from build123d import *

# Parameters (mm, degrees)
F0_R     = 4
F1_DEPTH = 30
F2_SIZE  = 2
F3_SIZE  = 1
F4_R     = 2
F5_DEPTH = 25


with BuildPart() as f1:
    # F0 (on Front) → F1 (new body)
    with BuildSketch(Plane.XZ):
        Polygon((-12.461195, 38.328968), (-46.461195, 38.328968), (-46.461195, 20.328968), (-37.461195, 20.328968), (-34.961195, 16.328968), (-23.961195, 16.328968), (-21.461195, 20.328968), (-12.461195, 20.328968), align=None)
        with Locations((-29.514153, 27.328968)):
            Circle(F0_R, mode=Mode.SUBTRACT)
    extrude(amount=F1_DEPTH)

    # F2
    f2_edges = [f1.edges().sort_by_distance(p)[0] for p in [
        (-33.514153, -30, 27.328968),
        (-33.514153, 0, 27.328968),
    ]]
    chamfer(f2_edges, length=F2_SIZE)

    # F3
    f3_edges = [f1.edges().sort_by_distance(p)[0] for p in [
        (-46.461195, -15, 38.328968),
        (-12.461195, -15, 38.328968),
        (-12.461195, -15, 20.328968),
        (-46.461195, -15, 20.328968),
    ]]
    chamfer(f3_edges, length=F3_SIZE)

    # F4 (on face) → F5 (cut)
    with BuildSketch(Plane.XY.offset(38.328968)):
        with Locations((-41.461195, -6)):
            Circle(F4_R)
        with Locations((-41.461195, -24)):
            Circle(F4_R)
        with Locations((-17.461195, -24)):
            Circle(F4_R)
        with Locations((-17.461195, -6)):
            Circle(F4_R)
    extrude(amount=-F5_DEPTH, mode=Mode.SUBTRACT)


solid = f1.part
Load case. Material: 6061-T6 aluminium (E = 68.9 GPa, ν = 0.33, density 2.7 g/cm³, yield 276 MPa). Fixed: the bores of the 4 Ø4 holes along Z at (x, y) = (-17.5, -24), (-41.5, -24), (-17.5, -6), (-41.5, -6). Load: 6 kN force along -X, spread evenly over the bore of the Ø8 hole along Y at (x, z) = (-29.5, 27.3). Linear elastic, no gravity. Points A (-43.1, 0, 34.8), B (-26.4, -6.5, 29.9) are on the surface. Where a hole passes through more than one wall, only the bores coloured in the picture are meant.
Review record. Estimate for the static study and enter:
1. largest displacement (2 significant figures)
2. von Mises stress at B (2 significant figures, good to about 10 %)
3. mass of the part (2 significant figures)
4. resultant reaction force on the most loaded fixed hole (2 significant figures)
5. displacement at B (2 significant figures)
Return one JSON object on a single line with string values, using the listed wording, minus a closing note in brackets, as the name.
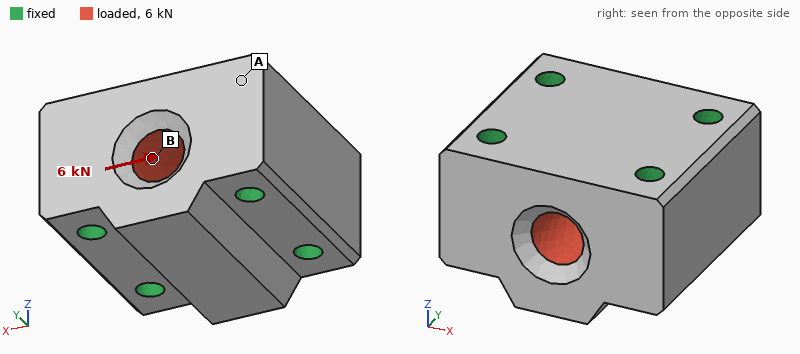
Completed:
{"largest displacement": "1.7 µm", "von Mises stress at B": "11 MPa", "mass of the part": "47 g", "resultant reaction force on the most loaded fixed hole": "1.5 kN", "displacement at B": "1.0 µm"}
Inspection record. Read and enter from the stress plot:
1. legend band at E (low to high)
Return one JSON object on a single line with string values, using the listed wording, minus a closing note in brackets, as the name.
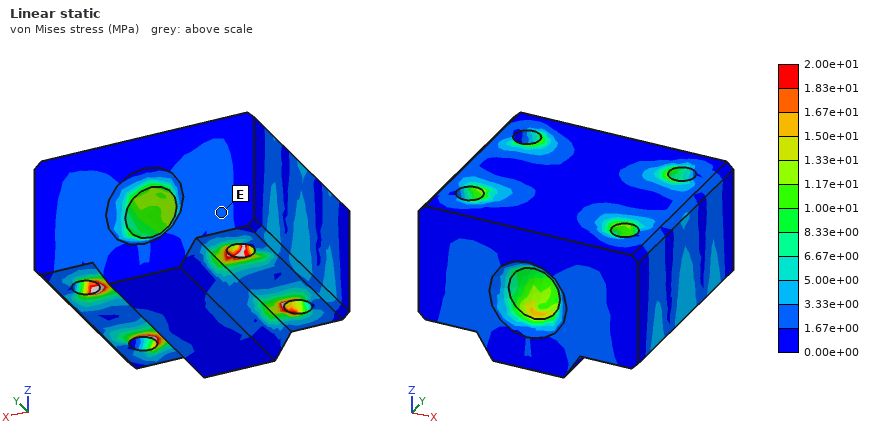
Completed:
{"legend band at E": "1.67e+00 to 3.33e+00 MPa"}
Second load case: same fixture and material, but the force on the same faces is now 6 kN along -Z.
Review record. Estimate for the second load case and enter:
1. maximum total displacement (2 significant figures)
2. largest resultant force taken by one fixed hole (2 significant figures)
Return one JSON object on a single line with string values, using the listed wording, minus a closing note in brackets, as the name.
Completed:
{"maximum total displacement": "3.2 µm", "largest resultant force taken by one fixed hole": "1.5 kN"}
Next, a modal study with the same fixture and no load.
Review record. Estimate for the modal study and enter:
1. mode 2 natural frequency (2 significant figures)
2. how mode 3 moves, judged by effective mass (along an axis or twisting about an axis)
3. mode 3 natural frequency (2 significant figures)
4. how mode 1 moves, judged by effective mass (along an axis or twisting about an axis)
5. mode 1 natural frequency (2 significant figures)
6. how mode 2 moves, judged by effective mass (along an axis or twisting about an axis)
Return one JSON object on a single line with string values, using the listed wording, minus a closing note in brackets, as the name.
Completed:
{"mode 2 natural frequency": "56 kHz", "how mode 3 moves, judged by effective mass": "along Y", "mode 3 natural frequency": "64 kHz", "how mode 1 moves, judged by effective mass": "along Y", "mode 1 natural frequency": "52 kHz", "how mode 2 moves, judged by effective mass": "along Z"}
